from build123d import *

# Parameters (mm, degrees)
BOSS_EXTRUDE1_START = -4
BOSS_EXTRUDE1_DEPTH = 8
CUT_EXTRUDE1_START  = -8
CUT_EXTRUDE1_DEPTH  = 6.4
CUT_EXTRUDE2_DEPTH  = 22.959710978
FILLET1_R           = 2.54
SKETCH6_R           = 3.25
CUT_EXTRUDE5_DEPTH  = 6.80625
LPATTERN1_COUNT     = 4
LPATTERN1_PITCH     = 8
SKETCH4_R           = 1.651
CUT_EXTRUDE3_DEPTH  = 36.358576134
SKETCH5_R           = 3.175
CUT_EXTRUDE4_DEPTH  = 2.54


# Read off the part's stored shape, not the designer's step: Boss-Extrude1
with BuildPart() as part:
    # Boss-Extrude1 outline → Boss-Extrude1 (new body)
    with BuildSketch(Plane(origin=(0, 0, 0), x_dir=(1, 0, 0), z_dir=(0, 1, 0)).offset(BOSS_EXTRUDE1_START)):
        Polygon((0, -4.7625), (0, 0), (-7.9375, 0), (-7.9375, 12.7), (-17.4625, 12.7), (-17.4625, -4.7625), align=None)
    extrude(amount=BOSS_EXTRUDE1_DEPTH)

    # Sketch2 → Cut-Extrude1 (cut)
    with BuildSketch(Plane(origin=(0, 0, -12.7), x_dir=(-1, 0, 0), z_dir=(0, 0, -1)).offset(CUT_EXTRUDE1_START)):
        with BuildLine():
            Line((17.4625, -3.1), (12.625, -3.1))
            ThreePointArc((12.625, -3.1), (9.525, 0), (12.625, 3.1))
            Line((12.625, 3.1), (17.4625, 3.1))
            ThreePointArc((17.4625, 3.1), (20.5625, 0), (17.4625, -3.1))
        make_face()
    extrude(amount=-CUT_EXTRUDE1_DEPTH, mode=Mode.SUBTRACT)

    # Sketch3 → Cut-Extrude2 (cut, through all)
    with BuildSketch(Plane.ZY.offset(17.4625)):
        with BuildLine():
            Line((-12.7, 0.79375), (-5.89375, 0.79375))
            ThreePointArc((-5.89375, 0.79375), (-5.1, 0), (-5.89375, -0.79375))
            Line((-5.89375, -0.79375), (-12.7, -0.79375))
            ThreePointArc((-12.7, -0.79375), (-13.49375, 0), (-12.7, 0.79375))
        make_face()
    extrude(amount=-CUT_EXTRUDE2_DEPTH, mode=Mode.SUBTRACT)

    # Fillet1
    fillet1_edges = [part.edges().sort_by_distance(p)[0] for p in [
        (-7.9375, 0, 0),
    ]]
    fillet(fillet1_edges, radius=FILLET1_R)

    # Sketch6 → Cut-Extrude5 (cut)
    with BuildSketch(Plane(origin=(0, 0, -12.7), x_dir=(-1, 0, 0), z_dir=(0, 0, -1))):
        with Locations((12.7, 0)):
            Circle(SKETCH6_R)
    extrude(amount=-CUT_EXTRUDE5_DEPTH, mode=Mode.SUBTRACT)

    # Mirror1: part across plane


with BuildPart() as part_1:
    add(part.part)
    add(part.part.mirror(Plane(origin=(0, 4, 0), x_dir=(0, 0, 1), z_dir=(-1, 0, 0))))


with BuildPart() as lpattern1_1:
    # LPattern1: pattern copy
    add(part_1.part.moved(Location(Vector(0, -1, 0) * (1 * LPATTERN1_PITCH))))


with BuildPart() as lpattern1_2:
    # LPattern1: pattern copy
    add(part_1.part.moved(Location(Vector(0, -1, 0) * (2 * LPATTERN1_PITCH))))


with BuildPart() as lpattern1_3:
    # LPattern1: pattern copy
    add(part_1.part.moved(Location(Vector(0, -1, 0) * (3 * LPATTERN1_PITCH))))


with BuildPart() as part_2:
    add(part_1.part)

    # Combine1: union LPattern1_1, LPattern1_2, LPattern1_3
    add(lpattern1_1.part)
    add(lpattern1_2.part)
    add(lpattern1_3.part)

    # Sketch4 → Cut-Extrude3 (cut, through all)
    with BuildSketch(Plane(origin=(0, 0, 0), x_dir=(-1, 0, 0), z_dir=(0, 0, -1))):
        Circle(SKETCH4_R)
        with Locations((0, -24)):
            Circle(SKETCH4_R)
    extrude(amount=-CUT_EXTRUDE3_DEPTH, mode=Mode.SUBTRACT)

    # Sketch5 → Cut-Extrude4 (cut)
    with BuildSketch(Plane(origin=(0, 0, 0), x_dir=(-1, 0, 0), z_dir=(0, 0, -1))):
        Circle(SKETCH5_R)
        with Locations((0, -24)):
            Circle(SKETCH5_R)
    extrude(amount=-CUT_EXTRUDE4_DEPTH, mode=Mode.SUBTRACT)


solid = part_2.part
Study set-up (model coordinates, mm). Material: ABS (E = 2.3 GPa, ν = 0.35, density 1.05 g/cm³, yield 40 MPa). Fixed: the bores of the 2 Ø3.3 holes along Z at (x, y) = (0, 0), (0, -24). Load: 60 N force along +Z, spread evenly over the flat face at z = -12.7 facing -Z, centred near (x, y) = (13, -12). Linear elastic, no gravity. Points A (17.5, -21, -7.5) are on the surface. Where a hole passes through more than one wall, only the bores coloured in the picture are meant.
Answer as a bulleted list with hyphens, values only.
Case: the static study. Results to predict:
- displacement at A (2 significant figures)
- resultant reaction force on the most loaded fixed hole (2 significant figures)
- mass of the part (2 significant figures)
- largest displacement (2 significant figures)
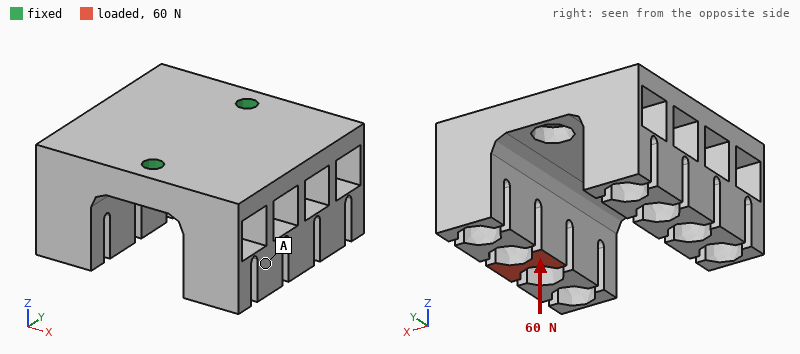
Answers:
- 0.35 mm
- 36 N
- 8.9 g
- 0.46 mm
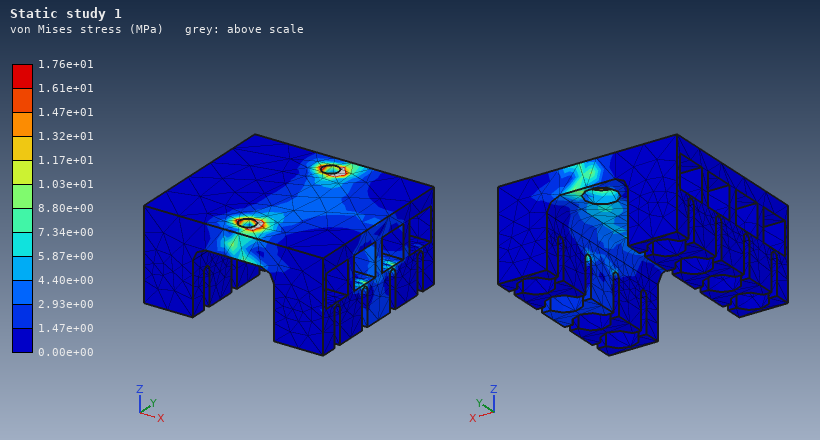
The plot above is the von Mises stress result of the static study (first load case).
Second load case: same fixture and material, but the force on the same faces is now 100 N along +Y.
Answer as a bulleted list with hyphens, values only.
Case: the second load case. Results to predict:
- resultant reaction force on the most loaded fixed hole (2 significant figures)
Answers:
- 99 N
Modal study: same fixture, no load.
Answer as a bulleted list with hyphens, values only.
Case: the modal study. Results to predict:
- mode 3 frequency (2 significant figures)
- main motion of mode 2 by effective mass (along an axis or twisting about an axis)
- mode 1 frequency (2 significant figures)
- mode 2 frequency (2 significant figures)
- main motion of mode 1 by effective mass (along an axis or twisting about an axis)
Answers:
- 2600 Hz
- along Z
- 940 Hz
- 1900 Hz
- along X
